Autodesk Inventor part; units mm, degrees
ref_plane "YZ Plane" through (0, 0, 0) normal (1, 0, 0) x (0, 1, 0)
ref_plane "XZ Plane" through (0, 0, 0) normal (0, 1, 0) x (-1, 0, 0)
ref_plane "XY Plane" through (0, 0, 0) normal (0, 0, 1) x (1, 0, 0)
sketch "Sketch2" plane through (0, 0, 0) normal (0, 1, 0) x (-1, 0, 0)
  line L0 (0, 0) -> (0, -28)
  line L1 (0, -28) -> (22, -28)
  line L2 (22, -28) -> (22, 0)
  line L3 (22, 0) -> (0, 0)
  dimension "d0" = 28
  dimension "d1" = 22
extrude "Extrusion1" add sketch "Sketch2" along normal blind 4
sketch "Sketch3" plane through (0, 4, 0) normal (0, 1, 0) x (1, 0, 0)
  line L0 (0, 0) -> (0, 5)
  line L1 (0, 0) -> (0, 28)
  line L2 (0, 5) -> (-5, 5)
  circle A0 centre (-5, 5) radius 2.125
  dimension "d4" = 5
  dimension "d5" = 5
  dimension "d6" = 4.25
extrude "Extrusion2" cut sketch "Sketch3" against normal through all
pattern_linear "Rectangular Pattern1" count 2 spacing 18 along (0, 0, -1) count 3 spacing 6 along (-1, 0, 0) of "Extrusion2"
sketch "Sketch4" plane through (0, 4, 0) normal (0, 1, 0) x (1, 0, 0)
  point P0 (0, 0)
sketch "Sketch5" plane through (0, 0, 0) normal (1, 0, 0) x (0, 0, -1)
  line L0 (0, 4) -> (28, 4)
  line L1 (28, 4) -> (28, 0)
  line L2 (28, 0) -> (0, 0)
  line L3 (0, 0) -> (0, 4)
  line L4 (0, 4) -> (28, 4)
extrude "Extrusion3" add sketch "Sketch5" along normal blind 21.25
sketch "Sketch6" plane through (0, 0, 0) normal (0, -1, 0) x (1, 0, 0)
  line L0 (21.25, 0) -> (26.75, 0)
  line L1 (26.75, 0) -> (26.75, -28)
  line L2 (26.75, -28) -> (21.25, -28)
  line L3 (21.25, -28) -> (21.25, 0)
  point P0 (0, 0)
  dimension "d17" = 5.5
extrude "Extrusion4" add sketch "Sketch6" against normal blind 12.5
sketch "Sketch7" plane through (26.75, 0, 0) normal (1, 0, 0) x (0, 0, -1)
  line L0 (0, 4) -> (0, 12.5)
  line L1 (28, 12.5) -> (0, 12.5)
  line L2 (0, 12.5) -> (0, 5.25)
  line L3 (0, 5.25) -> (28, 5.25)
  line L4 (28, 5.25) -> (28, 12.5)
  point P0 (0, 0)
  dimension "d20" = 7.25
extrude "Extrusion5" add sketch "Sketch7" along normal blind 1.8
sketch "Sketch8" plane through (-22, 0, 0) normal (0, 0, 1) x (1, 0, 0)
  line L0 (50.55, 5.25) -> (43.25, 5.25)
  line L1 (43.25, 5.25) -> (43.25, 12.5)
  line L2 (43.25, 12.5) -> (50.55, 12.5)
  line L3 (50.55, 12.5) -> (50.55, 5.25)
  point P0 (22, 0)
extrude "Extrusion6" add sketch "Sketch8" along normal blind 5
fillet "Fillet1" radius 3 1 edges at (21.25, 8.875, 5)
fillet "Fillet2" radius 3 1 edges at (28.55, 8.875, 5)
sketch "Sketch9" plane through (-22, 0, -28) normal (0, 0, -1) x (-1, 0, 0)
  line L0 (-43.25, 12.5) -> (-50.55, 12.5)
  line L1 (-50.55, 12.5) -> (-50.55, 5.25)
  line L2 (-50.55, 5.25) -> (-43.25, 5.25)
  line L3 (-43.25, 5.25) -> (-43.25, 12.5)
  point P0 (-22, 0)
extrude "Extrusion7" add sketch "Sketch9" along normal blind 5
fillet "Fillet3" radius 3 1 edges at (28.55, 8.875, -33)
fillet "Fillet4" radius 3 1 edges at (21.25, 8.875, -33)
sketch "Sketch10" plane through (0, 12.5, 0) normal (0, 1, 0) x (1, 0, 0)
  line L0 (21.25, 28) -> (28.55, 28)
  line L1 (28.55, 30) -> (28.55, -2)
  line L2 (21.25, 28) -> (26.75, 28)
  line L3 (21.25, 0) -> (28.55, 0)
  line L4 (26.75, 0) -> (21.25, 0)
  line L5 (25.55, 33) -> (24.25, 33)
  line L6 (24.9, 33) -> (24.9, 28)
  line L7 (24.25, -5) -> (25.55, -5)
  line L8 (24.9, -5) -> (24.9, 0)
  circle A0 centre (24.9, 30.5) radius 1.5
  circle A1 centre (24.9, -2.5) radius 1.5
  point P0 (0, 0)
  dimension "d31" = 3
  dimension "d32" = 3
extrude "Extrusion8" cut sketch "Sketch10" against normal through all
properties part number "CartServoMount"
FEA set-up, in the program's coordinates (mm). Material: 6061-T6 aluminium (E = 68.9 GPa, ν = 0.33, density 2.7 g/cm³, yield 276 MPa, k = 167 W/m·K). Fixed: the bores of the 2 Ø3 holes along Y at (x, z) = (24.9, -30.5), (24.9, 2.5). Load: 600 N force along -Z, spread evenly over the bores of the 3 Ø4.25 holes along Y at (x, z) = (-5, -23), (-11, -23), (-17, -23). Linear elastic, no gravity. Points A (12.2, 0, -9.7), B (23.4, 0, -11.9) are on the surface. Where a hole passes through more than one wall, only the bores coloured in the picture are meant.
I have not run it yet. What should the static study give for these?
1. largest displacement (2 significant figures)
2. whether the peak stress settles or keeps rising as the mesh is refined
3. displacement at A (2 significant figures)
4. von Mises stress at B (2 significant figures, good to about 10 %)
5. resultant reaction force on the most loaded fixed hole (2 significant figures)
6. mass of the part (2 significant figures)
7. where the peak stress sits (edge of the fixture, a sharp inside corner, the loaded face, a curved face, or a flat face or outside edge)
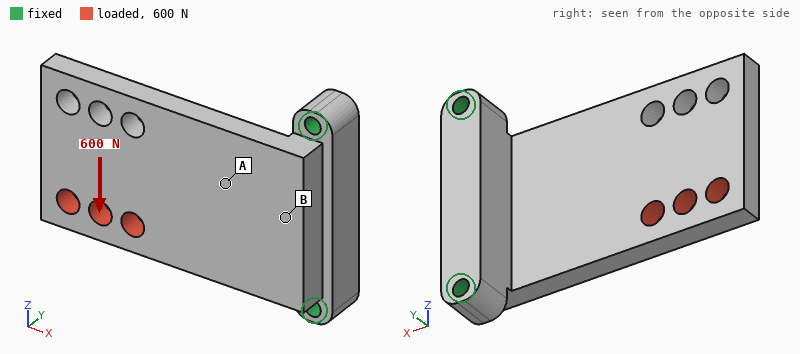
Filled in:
95 µm
keeps rising
18 µm
30 MPa
820 N
19 g
edge of the fixture
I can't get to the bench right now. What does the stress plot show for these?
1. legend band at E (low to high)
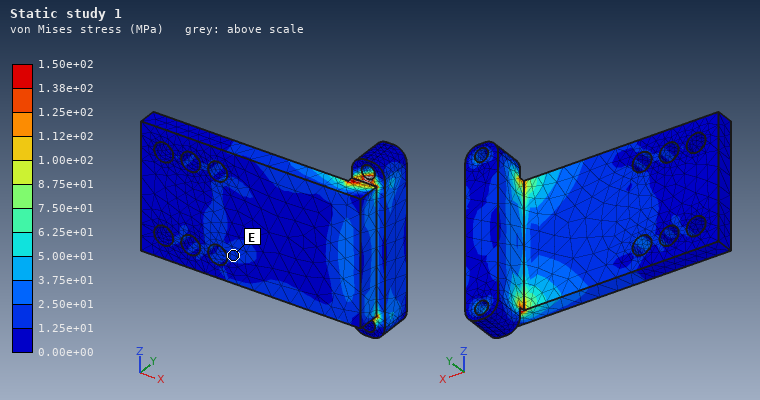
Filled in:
1.25e+01 to 2.50e+01 MPa
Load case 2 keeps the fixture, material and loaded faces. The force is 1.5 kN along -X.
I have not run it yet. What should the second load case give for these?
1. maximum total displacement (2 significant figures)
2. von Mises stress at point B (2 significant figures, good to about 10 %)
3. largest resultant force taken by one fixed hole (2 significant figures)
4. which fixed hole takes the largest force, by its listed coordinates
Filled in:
0.18 mm
26 MPa
1.2 kN
(24.9, -30.5)
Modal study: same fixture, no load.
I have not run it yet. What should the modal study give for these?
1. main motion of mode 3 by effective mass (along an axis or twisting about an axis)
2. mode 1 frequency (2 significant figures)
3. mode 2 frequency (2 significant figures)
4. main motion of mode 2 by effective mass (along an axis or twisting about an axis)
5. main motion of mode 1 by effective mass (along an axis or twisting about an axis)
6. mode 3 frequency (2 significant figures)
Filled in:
along Z
1500 Hz
5100 Hz
along Z
along Y
6100 Hz
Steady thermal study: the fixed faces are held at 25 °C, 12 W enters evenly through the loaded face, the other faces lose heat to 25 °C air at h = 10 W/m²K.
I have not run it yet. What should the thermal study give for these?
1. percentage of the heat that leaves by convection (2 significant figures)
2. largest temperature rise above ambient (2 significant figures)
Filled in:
5.0 %
33 K
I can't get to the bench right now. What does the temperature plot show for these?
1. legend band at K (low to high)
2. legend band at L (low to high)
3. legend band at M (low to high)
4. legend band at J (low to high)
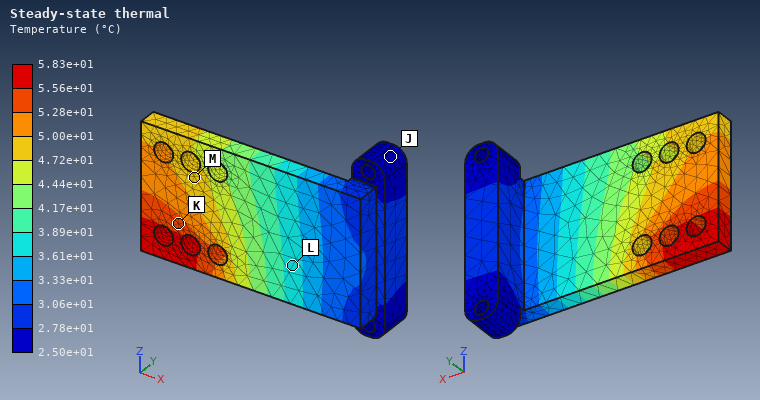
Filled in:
5.28e+01 to 5.56e+01 °C
3.61e+01 to 3.89e+01 °C
4.72e+01 to 5.00e+01 °C
2.50e+01 to 2.78e+01 °C
